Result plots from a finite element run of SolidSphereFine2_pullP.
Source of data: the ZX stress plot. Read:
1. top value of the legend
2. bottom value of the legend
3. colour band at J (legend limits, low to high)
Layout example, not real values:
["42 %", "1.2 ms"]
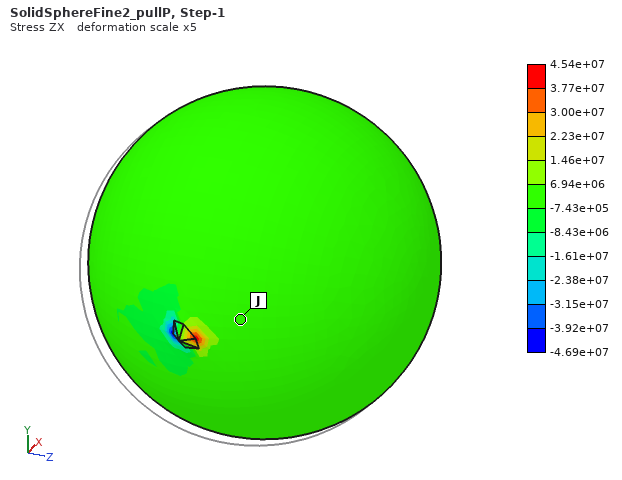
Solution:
["4.54e+07", "-4.69e+07", "-7.43e+05 to 6.94e+06"]
